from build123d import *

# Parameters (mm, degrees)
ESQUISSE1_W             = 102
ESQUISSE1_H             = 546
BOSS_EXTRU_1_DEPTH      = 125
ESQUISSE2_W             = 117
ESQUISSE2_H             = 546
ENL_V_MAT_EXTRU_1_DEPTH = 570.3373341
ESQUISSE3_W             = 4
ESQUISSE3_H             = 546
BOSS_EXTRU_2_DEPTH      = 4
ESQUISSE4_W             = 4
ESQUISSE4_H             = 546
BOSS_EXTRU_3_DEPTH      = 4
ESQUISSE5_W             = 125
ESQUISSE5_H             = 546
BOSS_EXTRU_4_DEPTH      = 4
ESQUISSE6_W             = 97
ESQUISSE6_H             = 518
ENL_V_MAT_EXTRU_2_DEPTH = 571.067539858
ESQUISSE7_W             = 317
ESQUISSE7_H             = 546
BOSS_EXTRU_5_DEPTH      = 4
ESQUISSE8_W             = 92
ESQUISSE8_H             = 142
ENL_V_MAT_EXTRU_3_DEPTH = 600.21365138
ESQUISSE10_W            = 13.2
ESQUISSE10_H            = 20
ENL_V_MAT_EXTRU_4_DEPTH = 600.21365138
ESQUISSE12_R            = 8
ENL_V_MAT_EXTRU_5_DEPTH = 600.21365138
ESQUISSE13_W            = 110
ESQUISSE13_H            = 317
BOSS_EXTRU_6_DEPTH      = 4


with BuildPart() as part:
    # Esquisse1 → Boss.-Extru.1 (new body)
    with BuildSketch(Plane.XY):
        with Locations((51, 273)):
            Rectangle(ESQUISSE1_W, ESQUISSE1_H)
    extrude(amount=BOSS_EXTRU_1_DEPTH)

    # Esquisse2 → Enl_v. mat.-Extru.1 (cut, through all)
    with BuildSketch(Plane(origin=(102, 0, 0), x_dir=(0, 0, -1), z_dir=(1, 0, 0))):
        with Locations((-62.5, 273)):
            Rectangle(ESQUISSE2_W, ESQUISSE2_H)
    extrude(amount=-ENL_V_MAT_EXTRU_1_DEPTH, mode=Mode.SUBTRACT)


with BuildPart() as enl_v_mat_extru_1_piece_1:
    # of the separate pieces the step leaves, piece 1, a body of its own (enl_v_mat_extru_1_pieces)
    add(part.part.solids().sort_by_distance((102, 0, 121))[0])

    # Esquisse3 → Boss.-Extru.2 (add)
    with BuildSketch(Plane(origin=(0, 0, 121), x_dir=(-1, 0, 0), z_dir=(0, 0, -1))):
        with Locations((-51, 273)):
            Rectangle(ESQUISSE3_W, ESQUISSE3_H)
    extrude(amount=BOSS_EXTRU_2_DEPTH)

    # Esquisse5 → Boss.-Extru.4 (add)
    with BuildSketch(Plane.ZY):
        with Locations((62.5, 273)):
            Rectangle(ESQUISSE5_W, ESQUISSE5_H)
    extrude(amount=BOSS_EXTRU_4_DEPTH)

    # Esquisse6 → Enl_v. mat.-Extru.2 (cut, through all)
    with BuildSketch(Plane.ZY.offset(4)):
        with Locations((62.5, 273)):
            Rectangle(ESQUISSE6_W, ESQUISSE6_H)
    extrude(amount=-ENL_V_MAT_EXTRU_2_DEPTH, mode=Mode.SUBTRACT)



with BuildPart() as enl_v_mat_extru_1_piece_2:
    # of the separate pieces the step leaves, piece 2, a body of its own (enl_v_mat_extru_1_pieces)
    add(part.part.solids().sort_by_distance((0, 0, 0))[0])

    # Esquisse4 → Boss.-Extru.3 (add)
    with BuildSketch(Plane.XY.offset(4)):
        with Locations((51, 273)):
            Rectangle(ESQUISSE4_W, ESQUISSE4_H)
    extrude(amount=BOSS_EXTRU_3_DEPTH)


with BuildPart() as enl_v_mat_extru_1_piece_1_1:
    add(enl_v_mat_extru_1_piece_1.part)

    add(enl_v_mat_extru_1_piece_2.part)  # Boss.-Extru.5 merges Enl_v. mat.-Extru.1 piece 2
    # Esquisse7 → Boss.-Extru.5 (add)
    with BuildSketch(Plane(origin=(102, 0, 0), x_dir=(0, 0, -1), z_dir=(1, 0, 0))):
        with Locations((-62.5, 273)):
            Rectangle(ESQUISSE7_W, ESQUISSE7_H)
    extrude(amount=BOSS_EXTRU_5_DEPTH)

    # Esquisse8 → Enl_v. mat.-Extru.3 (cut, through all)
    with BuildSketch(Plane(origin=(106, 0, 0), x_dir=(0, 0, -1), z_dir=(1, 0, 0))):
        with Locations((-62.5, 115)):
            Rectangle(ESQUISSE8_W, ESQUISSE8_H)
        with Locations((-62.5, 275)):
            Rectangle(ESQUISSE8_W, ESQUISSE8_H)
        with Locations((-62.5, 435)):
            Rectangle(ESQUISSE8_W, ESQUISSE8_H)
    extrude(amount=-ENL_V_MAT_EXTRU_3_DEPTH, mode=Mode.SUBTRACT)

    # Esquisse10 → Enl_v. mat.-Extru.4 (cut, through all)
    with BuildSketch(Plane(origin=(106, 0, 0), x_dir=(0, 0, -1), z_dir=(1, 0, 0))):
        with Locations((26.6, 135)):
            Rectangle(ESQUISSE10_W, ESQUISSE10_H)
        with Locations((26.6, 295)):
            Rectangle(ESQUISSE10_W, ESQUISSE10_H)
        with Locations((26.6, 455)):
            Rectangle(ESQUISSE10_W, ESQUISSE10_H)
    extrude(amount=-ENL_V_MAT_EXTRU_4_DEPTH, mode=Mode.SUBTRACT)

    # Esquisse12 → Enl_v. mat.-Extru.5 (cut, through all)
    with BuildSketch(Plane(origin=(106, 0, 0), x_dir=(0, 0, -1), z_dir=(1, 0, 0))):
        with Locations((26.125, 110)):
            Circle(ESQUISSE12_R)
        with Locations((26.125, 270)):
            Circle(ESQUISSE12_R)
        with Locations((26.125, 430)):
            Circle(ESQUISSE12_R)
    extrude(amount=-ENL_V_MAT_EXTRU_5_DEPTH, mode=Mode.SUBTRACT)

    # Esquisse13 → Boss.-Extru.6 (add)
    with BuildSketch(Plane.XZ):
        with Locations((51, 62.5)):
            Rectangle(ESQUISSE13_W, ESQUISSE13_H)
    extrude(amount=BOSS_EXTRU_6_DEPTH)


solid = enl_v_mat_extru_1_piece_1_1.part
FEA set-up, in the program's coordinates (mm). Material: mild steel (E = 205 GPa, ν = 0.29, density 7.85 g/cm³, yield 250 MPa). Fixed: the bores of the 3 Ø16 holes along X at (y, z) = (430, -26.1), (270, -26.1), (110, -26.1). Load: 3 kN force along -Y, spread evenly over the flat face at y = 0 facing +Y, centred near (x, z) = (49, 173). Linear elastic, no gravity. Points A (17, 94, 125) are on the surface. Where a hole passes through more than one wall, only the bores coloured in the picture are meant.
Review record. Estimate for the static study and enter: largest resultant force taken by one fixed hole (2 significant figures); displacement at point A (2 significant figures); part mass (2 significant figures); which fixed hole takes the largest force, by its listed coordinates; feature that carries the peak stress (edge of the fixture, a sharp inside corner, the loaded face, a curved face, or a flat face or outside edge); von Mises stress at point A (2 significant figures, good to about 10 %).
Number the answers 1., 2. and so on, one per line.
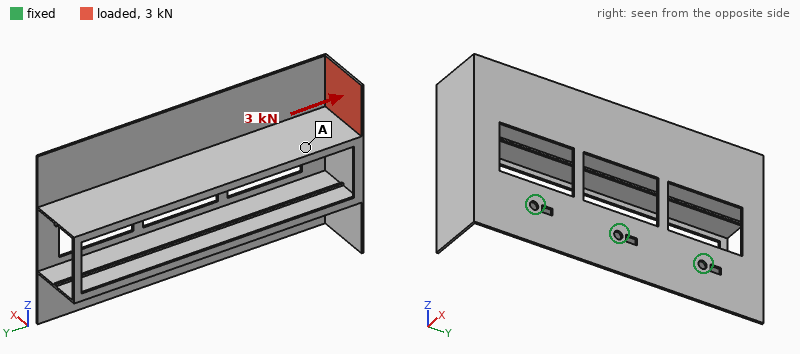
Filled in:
1. 2.4 kN
2. 0.48 mm
3. 9.5 kg
4. (110, -26.1)
5. a flat face or outside edge
6. 21 MPa
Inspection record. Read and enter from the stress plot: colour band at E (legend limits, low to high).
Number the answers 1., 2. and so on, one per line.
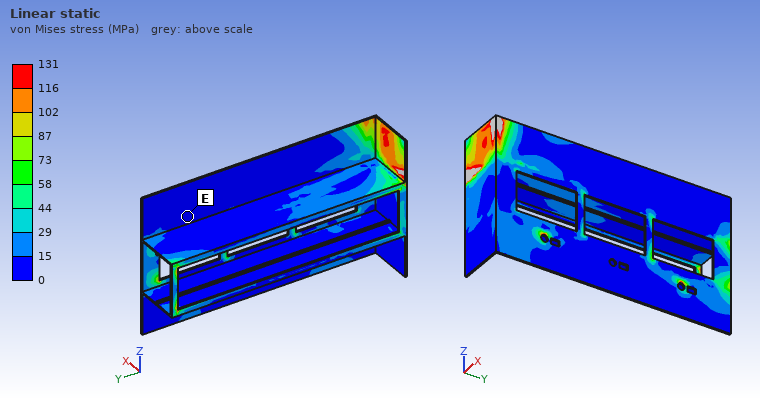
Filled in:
1. 0 to 15 MPa
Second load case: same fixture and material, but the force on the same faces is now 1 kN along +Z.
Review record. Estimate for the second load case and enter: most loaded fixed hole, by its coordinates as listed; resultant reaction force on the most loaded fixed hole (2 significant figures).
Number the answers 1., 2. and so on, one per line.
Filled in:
1. (110, -26.1)
2. 1.4 kN
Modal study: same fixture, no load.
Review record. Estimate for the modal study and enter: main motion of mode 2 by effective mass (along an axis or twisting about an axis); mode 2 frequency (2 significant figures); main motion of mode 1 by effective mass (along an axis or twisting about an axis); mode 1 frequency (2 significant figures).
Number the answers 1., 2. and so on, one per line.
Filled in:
1. twisting about Z
2. 87 Hz
3. along X
4. 40 Hz
